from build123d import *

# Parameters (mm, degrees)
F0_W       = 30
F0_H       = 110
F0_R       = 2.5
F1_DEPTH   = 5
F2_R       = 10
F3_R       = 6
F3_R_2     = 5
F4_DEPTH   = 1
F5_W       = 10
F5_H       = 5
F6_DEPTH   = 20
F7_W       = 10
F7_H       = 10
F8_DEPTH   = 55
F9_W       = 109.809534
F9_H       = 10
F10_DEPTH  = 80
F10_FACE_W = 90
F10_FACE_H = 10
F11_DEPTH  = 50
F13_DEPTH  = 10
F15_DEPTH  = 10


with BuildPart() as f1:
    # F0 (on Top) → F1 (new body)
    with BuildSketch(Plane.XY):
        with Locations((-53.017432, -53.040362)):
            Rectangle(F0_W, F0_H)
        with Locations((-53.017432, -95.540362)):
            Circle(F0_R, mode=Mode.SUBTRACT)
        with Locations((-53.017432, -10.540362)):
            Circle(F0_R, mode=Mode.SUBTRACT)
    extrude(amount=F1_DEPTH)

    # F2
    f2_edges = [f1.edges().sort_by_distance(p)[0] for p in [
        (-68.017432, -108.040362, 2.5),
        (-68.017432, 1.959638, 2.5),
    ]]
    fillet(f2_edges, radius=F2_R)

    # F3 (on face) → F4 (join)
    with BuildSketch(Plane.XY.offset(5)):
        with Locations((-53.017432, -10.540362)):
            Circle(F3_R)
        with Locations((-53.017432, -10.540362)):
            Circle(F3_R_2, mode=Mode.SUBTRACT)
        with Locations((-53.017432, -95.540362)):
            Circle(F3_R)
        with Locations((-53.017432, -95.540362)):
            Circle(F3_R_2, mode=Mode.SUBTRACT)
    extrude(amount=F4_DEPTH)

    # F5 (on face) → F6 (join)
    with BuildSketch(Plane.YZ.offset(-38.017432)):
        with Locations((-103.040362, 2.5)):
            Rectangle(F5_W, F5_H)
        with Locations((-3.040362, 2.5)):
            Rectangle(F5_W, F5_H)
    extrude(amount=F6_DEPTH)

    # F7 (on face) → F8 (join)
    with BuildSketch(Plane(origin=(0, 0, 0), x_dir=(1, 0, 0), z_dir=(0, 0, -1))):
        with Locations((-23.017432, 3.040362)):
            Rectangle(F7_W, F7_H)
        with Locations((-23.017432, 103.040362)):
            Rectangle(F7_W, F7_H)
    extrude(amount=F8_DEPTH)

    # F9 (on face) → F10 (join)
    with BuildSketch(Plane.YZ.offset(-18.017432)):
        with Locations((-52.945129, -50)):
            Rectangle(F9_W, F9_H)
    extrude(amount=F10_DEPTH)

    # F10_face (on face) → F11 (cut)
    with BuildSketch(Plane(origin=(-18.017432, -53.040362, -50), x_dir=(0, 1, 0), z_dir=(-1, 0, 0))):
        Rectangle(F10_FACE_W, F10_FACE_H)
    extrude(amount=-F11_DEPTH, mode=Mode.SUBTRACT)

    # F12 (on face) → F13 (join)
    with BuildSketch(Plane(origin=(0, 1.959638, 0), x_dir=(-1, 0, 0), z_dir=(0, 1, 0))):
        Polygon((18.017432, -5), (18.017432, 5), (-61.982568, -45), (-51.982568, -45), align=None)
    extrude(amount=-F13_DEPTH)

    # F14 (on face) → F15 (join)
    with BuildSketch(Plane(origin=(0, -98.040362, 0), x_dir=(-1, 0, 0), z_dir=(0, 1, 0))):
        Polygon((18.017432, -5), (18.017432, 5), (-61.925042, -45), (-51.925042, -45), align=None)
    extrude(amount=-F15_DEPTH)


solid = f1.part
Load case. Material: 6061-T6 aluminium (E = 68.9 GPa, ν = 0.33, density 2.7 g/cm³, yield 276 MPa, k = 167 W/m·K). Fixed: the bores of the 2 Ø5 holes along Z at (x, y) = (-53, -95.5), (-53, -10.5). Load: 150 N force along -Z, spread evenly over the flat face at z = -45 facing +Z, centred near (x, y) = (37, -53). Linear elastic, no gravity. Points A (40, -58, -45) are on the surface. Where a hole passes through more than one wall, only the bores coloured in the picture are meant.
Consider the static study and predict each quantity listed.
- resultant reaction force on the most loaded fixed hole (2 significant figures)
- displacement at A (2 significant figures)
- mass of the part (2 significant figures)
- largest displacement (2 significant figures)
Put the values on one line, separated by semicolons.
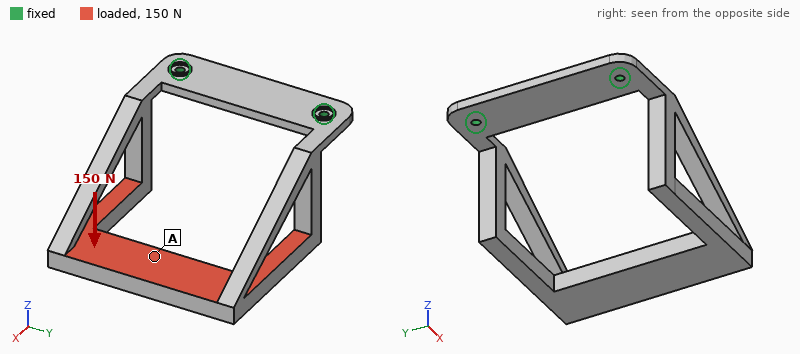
75 N; 1.6 mm; 230 g; 2.0 mm
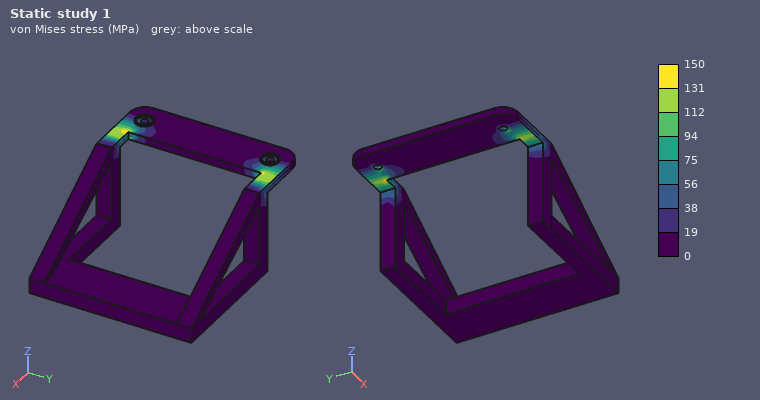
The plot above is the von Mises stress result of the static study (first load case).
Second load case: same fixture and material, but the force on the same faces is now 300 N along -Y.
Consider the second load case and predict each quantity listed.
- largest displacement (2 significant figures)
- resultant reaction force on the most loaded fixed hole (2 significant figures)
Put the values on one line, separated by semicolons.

0.45 mm; 340 N
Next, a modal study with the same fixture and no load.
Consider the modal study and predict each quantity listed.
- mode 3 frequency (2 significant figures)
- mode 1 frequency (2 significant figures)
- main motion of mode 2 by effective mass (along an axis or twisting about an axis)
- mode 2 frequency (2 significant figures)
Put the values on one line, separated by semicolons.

540 Hz; 120 Hz; along Y; 350 Hz
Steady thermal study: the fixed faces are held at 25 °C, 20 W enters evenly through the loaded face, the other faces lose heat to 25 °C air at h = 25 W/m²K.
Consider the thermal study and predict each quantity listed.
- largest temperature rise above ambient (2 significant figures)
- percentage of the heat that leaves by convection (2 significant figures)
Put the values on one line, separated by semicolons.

33 K; 59 %
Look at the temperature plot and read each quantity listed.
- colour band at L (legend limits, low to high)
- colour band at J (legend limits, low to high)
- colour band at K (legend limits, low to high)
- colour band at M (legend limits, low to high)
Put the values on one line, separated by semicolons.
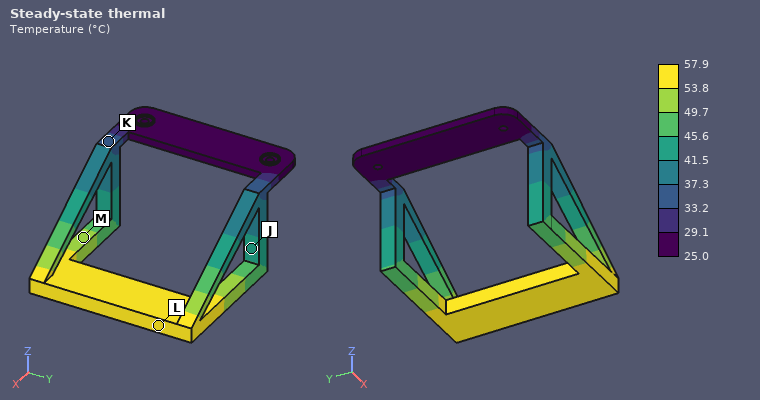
53.8 to 57.9 °C; 41.5 to 45.6 °C; 33.2 to 37.3 °C; 49.7 to 53.8 °C
